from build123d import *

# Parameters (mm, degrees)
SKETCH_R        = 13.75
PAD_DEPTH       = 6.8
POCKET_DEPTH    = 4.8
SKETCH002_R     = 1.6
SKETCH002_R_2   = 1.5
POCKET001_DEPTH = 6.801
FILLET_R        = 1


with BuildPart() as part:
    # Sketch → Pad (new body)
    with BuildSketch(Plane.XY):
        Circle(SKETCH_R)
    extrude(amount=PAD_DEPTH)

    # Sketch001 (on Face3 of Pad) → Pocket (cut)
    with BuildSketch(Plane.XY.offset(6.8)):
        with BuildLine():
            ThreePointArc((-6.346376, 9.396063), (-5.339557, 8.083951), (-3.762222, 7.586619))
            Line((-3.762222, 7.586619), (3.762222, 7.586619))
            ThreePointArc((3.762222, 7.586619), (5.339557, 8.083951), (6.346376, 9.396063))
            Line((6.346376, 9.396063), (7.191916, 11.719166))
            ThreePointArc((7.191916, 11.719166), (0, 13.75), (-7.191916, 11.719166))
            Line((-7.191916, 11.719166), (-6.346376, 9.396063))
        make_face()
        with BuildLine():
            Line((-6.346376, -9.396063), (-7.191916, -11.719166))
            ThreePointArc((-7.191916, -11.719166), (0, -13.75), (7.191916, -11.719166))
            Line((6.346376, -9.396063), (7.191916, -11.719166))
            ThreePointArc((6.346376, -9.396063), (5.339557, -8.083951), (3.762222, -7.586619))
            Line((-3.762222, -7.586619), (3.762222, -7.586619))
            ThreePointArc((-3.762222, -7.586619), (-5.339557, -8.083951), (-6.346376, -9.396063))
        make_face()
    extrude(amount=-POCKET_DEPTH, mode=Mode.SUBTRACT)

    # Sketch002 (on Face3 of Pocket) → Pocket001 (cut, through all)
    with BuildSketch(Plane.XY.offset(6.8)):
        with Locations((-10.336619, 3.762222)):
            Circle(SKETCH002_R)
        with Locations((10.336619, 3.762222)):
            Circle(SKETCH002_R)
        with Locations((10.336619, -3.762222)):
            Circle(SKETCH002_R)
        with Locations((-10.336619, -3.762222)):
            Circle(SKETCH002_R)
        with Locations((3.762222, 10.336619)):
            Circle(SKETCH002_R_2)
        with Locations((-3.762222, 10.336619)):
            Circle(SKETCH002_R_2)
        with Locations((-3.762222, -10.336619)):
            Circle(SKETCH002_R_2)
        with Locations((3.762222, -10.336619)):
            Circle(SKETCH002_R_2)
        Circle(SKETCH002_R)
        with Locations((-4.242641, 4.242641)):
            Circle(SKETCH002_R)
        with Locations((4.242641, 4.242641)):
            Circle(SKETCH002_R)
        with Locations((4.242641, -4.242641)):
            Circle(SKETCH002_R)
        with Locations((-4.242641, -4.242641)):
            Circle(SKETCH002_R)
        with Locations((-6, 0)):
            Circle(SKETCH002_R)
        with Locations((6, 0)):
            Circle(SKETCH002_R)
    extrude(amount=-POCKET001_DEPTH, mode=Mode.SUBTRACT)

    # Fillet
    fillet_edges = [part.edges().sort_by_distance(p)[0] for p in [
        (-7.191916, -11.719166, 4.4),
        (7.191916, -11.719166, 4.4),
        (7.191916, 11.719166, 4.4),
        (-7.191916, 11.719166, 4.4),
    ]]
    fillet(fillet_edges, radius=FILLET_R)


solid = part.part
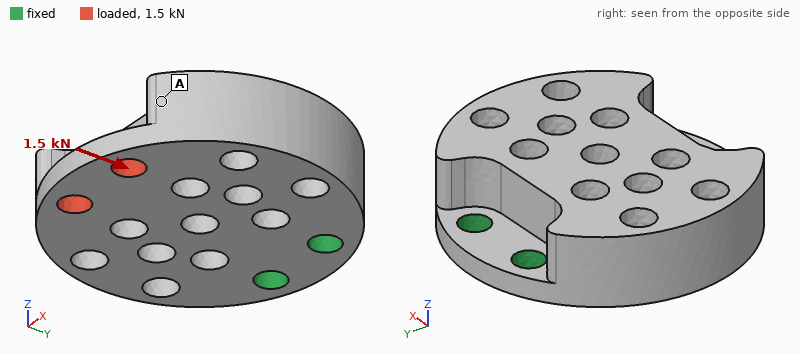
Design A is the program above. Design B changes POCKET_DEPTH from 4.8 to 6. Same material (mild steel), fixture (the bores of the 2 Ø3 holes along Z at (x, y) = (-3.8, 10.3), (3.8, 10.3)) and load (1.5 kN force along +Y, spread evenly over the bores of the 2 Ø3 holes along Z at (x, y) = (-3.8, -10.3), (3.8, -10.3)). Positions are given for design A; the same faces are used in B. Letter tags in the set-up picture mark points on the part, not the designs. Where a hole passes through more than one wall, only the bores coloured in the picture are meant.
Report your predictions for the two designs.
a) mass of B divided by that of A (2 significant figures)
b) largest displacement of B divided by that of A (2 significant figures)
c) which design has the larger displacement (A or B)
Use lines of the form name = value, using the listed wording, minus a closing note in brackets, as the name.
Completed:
mass of B divided by that of A = 0.95
largest displacement of B divided by that of A = 1.3
which design has the larger displacement = B
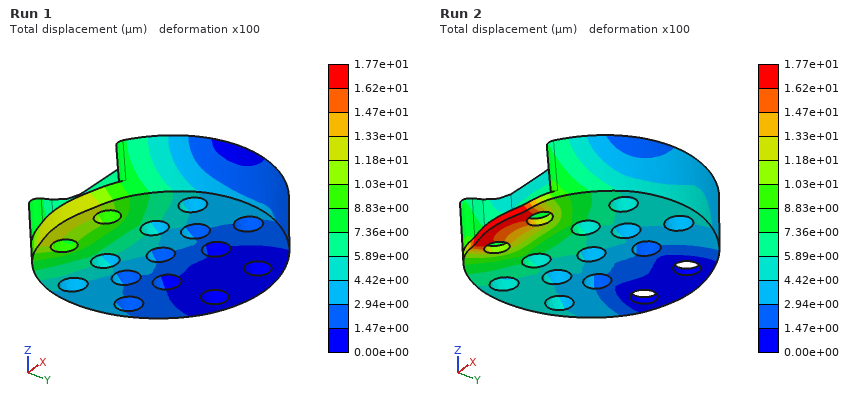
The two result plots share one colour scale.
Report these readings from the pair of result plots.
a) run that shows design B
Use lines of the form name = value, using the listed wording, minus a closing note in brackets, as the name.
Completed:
run that shows design B = Run 2
